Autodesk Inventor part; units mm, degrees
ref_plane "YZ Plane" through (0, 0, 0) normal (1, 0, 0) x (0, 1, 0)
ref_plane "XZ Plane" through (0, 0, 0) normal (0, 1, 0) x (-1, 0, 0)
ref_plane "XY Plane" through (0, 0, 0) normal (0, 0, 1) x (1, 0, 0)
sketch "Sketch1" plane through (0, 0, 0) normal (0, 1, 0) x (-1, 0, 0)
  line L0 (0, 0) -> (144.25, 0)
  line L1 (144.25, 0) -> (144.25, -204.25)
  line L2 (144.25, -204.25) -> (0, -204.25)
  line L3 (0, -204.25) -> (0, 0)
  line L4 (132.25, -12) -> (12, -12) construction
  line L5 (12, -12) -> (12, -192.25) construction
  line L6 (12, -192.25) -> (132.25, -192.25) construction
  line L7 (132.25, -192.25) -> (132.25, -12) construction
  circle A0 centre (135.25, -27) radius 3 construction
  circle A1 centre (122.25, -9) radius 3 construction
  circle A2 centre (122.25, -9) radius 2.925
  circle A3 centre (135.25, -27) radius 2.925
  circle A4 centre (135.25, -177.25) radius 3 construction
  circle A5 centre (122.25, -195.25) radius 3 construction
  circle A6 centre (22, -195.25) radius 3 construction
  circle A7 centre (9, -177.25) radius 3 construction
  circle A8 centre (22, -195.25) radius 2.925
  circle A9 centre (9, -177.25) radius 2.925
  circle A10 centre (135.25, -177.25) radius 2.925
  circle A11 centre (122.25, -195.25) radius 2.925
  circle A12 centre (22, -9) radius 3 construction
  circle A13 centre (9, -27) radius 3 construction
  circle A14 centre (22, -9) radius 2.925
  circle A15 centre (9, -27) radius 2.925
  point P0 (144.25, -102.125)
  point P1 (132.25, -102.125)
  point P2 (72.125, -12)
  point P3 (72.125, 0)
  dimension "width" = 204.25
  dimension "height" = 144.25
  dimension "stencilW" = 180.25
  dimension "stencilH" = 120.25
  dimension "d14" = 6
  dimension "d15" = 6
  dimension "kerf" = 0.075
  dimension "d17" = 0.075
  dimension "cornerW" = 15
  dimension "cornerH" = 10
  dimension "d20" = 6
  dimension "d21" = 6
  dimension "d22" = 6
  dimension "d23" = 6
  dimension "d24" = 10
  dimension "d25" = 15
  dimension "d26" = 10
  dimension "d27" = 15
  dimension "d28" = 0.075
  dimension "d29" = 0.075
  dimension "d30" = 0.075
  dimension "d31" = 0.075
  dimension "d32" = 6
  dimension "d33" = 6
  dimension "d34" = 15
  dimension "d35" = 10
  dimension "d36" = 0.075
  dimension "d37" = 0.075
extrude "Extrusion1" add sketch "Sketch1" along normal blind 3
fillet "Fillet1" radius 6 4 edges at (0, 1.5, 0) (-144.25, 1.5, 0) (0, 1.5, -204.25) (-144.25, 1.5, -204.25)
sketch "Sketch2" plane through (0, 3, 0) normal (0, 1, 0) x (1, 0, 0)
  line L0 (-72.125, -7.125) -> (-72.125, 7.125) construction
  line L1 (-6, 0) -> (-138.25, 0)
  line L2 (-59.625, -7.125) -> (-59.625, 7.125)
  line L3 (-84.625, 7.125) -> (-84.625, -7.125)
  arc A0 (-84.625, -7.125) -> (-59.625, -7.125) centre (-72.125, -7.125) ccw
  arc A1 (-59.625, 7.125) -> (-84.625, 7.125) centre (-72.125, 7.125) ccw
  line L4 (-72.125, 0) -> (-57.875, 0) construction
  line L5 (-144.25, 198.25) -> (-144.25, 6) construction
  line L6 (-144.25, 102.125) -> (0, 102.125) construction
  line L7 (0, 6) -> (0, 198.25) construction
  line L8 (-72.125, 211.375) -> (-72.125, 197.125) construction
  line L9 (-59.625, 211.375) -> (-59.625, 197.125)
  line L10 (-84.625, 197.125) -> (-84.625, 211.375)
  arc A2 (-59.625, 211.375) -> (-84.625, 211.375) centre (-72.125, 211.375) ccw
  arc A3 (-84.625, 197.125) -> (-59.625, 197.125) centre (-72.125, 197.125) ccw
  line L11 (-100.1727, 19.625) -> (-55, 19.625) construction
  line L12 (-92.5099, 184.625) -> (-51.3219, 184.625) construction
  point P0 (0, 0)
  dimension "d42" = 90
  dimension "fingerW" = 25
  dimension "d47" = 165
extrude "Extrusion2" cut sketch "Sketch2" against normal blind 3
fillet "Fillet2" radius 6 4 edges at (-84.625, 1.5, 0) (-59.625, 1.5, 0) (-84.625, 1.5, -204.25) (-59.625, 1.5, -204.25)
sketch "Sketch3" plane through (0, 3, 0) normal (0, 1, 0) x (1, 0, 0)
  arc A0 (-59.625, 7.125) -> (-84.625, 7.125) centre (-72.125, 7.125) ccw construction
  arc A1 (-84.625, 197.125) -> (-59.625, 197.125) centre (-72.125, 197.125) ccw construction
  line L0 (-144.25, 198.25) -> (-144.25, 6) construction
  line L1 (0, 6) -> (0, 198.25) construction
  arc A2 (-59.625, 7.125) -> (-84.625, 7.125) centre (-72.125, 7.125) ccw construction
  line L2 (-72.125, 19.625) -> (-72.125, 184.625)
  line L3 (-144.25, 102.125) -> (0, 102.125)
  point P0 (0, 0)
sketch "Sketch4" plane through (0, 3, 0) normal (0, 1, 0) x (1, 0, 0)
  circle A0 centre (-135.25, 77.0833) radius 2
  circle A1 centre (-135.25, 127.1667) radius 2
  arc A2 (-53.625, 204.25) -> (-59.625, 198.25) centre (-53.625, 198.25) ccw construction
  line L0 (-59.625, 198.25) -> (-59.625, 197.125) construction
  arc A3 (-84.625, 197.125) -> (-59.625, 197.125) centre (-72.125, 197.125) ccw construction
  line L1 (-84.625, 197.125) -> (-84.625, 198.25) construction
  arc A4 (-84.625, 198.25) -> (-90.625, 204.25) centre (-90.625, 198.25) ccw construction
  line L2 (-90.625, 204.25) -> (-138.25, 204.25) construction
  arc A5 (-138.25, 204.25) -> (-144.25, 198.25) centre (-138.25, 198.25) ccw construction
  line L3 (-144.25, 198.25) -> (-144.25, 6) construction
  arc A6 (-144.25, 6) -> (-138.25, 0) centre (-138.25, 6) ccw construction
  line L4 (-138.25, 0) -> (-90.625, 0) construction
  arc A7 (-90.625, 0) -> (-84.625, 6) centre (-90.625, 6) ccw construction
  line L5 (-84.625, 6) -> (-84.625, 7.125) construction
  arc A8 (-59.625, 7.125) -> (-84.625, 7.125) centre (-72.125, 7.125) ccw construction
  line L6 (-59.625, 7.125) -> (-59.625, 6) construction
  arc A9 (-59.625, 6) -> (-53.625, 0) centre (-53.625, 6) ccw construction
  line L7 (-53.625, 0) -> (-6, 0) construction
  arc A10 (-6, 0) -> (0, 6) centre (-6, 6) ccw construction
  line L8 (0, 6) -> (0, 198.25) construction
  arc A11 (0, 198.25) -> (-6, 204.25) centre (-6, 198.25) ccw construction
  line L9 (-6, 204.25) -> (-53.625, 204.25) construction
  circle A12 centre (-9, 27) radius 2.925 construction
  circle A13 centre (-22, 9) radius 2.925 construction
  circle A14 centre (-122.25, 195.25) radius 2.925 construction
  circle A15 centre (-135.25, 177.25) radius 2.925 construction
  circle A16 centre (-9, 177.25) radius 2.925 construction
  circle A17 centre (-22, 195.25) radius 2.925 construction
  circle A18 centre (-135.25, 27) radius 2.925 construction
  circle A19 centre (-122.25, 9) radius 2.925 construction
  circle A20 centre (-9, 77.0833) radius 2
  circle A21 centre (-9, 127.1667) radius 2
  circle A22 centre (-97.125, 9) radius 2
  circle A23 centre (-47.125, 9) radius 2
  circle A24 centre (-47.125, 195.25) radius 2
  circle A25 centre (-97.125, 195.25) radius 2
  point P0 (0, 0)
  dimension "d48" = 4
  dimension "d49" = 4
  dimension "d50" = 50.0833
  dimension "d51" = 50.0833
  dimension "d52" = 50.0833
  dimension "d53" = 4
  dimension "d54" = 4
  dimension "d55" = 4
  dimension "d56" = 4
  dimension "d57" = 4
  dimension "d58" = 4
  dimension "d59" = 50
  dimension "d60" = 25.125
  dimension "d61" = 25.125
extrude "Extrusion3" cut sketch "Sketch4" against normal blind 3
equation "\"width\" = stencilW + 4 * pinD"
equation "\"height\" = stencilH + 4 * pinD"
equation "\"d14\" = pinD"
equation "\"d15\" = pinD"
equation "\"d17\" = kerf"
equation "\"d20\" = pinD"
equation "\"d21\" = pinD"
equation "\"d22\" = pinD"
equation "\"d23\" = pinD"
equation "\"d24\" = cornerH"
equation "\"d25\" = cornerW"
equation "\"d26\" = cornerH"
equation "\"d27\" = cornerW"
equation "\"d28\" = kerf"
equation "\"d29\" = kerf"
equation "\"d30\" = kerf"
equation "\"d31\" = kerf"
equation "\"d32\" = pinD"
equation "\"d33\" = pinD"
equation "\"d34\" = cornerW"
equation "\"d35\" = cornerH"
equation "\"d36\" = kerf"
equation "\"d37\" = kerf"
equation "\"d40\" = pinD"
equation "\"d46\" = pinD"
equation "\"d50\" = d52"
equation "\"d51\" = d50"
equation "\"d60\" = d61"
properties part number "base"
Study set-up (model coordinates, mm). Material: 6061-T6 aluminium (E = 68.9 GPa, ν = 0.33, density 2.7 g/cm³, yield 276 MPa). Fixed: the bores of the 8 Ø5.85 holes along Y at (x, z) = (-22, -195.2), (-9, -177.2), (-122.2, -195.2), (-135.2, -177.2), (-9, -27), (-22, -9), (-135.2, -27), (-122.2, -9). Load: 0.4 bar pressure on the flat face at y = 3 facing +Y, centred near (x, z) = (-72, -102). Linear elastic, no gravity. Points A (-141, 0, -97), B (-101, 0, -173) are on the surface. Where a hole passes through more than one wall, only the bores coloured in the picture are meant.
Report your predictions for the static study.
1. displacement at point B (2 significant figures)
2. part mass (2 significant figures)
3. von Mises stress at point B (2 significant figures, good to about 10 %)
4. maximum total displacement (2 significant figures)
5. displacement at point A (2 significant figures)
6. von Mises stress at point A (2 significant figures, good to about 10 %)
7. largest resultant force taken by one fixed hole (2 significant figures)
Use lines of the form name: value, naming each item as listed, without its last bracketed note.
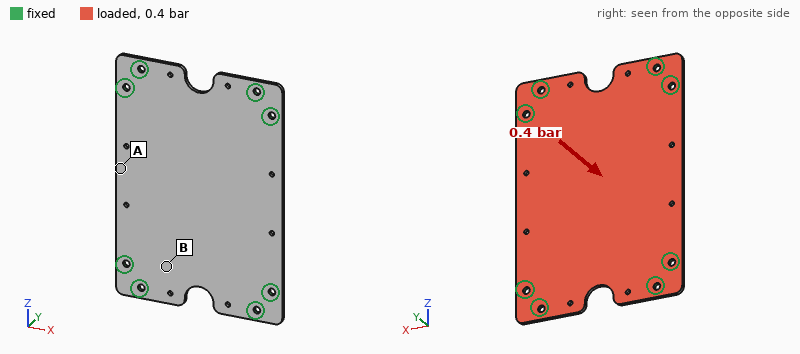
displacement at point B: 0.16 mm
part mass: 230 g
von Mises stress at point B: 16 MPa
maximum total displacement: 0.62 mm
displacement at point A: 0.45 mm
von Mises stress at point A: 33 MPa
largest resultant force taken by one fixed hole: 240 N
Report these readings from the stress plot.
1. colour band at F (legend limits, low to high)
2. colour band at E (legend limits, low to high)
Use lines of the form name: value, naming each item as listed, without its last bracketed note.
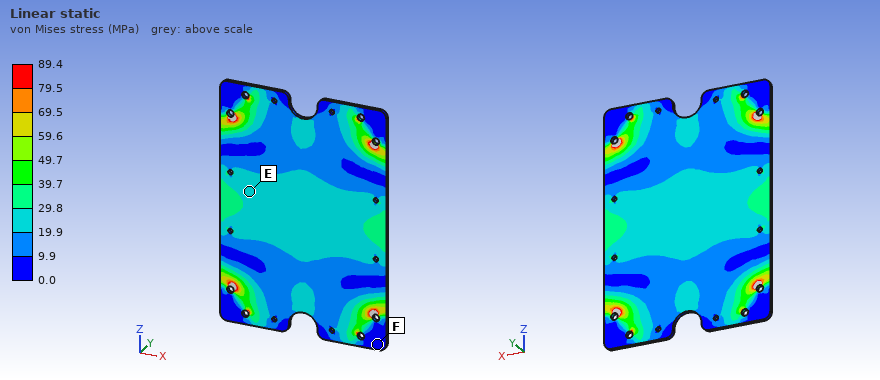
colour band at F: 0.0 to 9.9 MPa
colour band at E: 19.9 to 29.8 MPa
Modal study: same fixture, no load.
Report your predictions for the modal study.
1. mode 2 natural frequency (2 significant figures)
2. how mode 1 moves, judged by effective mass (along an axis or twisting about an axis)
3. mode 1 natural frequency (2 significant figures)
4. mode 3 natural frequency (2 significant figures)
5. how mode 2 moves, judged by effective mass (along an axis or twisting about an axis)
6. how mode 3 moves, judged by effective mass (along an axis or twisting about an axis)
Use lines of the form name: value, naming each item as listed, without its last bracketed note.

mode 2 natural frequency: 840 Hz
how mode 1 moves, judged by effective mass: along Y
mode 1 natural frequency: 540 Hz
mode 3 natural frequency: 1200 Hz
how mode 2 moves, judged by effective mass: twisting about Z
how mode 3 moves, judged by effective mass: twisting about X
